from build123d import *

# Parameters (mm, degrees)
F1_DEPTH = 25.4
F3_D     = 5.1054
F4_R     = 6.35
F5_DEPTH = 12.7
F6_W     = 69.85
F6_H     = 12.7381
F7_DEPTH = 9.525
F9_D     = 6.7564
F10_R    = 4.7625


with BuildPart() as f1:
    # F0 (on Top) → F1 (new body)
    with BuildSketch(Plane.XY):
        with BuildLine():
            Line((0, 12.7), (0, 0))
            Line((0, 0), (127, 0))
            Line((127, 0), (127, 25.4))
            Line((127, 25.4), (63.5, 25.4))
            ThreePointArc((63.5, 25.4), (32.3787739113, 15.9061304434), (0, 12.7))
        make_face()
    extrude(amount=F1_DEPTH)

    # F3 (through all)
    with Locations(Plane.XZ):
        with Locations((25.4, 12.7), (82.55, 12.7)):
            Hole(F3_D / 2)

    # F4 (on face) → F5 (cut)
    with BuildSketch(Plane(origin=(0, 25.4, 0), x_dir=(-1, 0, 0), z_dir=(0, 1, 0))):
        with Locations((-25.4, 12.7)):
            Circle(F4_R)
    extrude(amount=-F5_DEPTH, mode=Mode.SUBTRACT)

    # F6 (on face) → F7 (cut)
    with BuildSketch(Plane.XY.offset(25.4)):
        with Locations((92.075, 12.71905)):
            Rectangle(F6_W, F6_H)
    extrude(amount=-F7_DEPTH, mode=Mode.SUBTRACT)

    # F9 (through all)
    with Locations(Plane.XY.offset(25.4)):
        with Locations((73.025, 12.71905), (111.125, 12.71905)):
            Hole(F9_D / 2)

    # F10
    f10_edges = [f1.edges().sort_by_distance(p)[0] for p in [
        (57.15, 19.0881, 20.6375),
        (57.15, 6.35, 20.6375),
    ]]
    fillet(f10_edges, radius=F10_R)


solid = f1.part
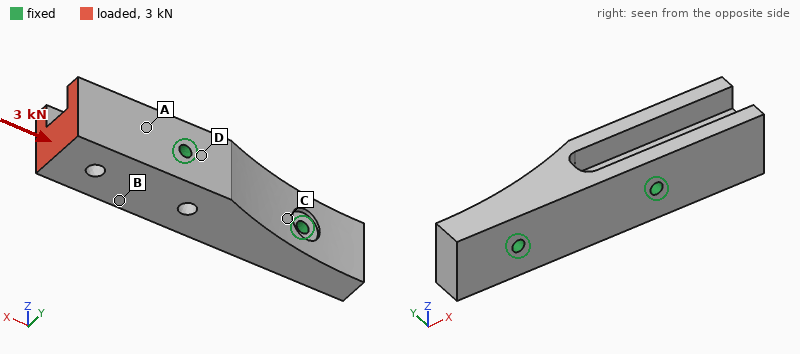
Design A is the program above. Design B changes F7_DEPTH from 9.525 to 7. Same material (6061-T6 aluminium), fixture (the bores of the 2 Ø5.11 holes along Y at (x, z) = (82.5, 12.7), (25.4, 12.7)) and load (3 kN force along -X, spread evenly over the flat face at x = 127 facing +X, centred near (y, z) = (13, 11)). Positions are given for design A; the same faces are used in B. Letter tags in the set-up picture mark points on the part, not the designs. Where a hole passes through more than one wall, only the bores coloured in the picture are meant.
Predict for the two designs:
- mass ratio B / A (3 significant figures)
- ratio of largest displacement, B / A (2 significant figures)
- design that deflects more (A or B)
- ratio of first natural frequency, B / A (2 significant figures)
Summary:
1.04
0.91
A
1.0
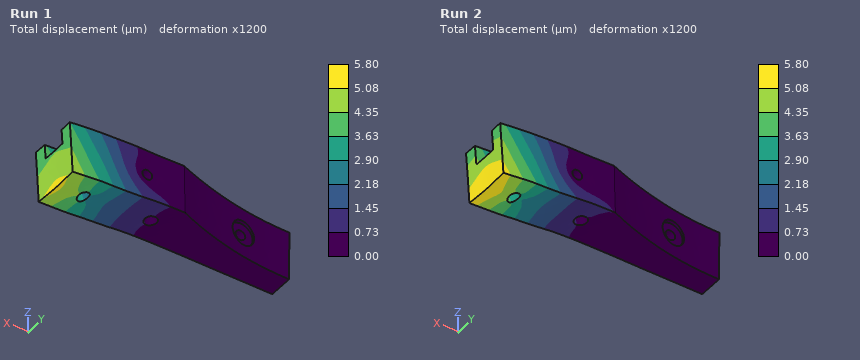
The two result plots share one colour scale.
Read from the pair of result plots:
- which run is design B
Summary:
Run 1
